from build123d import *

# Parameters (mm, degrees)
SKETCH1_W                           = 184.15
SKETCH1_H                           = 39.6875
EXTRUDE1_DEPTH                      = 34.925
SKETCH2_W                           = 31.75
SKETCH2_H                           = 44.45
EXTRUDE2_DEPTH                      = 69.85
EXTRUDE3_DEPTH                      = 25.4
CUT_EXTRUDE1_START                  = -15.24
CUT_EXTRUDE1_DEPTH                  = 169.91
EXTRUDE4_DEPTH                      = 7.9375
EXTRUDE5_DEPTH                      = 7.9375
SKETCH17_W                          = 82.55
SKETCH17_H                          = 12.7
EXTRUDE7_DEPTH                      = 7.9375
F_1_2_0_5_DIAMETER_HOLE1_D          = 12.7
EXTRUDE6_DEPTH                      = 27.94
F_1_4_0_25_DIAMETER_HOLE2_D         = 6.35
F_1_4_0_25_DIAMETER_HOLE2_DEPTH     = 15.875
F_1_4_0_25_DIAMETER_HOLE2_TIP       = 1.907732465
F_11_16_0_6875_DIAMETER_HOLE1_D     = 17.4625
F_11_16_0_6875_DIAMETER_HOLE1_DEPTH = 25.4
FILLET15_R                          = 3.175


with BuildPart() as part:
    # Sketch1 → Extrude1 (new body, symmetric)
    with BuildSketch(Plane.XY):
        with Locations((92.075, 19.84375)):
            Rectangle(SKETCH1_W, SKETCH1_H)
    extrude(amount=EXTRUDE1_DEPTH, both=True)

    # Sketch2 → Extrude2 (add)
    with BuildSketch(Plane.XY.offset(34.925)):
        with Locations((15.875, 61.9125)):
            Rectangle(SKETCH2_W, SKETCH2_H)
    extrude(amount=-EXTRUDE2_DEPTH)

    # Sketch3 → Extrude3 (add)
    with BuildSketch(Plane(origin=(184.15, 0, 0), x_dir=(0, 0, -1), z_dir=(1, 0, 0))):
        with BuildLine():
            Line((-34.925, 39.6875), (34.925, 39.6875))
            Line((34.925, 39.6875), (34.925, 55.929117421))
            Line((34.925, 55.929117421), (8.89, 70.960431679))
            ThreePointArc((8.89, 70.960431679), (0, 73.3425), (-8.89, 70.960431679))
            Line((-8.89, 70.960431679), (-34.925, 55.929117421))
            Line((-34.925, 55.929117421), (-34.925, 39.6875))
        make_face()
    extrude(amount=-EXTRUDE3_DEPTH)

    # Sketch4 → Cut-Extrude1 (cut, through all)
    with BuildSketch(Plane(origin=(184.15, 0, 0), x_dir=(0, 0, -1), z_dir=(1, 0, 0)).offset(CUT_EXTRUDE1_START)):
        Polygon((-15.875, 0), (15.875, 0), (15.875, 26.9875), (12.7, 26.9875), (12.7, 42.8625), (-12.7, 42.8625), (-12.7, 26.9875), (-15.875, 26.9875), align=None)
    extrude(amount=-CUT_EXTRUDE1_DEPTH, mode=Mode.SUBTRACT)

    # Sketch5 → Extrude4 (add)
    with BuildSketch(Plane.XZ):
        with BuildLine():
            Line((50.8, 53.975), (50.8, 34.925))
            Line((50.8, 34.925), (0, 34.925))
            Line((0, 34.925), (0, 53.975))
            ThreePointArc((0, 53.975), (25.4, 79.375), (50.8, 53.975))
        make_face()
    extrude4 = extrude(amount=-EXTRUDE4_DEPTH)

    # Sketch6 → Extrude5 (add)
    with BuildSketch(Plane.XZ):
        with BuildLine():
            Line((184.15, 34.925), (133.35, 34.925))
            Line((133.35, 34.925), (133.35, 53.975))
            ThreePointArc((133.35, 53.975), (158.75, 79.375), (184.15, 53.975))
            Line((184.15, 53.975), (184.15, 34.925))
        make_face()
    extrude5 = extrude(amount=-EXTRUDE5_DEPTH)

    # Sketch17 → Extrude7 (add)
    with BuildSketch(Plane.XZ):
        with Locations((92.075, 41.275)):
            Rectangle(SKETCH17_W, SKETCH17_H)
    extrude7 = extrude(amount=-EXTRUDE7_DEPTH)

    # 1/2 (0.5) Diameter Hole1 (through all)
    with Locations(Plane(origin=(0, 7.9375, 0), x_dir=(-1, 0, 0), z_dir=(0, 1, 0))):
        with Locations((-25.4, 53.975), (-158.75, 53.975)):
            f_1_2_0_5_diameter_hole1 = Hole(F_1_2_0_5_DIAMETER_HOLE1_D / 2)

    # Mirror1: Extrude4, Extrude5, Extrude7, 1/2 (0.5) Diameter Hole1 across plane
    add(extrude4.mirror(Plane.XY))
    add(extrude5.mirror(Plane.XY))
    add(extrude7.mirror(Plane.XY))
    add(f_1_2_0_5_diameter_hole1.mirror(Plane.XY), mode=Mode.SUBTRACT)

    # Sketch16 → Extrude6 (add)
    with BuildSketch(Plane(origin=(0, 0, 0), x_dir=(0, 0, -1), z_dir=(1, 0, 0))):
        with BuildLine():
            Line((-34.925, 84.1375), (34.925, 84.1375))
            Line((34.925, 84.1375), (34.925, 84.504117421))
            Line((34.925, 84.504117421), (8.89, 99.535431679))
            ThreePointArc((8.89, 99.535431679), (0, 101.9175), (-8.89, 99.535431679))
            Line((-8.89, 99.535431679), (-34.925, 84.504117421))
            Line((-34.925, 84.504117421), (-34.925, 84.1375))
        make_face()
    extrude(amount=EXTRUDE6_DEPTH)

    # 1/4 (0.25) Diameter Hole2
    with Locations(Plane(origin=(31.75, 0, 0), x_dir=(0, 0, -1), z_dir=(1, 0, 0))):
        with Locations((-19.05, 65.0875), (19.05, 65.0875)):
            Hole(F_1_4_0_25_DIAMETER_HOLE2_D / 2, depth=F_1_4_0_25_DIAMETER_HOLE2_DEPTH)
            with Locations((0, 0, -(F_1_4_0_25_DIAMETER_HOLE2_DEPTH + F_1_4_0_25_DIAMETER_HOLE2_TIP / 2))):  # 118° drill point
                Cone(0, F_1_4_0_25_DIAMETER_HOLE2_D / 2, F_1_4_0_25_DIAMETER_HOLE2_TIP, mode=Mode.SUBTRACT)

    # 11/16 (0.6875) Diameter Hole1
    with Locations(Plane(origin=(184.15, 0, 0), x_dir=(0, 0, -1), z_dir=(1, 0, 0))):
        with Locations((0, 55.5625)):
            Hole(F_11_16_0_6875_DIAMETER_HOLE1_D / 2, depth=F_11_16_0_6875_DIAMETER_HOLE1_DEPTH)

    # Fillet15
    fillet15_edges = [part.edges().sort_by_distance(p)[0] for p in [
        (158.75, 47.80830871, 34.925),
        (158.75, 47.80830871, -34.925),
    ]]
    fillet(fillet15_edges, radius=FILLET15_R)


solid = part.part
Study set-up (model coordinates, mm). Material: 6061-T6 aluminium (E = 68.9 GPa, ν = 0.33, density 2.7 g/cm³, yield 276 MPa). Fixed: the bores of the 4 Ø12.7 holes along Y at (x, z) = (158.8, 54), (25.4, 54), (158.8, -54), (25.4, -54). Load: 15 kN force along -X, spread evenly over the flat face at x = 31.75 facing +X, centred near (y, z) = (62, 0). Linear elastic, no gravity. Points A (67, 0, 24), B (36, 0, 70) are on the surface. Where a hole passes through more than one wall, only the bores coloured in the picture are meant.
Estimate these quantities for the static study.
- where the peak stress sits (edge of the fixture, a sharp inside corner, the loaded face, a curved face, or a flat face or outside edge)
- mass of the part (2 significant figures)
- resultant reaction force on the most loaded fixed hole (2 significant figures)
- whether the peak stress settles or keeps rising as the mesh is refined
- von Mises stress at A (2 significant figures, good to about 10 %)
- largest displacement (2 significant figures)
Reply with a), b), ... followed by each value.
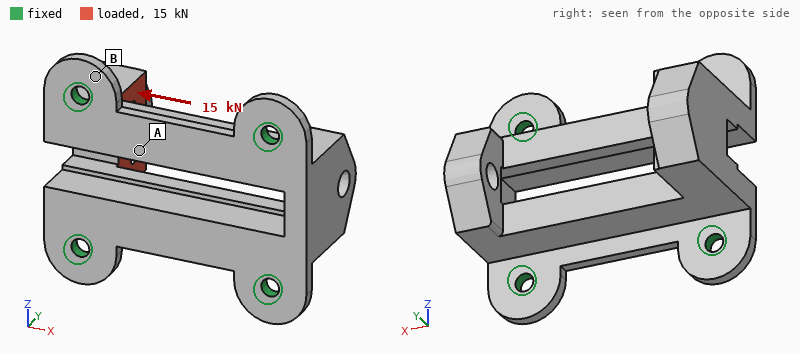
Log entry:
a) edge of the fixture
b) 1.5 kg
c) 6.3 kN
d) keeps rising
e) 21 MPa
f) 0.29 mm
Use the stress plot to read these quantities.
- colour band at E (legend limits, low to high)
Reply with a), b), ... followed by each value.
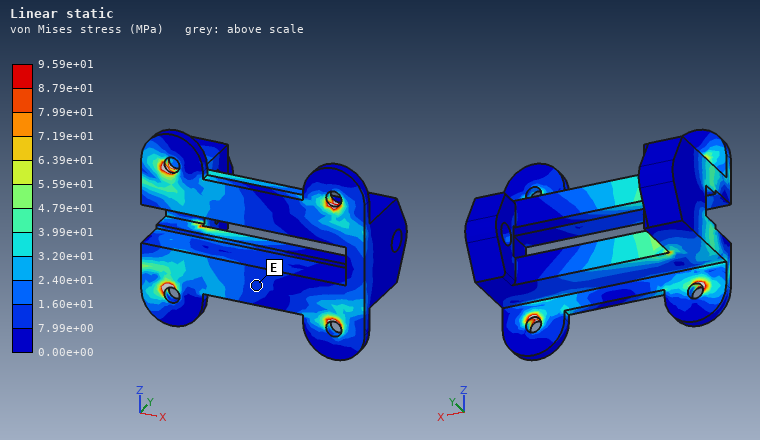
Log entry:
a) 7.99e+00 to 1.60e+01 MPa
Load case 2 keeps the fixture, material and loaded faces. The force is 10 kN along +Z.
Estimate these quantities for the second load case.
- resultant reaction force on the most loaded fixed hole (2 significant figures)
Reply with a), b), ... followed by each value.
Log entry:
a) 7.7 kN
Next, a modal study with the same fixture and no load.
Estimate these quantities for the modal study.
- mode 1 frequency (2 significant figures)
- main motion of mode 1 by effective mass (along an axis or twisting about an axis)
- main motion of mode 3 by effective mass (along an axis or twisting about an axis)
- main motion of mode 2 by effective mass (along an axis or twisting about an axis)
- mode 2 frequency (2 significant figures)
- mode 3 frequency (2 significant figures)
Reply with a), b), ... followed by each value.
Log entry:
a) 2100 Hz
b) along X
c) along Y
d) along Z
e) 2400 Hz
f) 2700 Hz
